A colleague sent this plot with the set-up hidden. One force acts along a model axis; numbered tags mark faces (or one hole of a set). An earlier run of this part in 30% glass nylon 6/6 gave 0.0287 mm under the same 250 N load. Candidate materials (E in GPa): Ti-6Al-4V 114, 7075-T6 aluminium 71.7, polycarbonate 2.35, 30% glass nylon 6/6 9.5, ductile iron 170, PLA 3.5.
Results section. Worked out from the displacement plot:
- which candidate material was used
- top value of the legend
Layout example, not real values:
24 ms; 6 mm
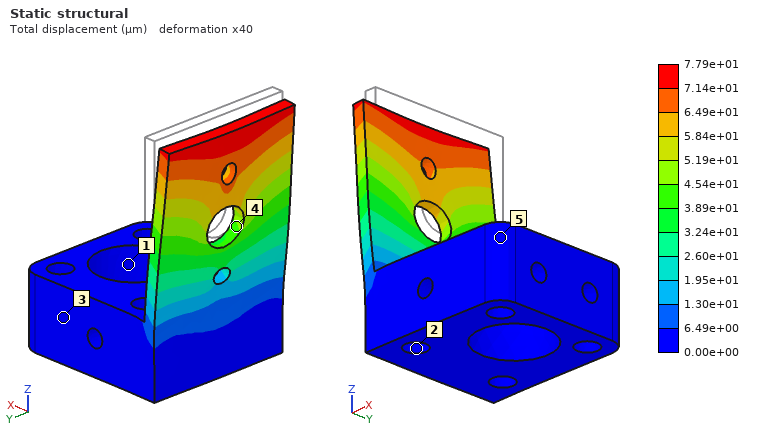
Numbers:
PLA; 7.79e+01 µm
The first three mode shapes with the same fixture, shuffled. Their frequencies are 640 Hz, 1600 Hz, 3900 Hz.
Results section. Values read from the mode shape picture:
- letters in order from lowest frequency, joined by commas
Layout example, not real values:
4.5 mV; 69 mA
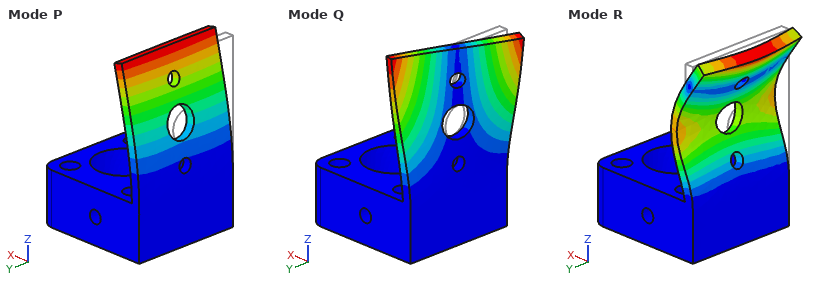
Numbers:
P, Q, R
